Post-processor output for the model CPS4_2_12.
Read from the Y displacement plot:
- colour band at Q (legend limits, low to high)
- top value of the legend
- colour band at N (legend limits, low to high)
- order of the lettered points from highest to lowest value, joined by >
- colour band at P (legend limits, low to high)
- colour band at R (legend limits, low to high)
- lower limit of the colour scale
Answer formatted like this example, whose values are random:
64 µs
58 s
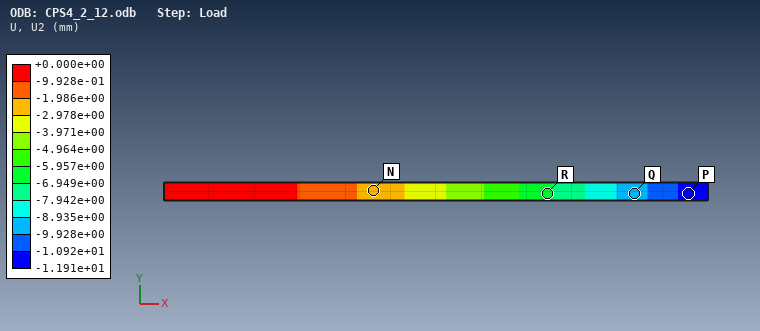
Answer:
-9.928e+00 to -8.935e+00 mm
+0.000e+00 mm
-2.978e+00 to -1.986e+00 mm
N > R > Q > P
-1.191e+01 to -1.092e+01 mm
-6.949e+00 to -5.957e+00 mm
-1.191e+01 mm
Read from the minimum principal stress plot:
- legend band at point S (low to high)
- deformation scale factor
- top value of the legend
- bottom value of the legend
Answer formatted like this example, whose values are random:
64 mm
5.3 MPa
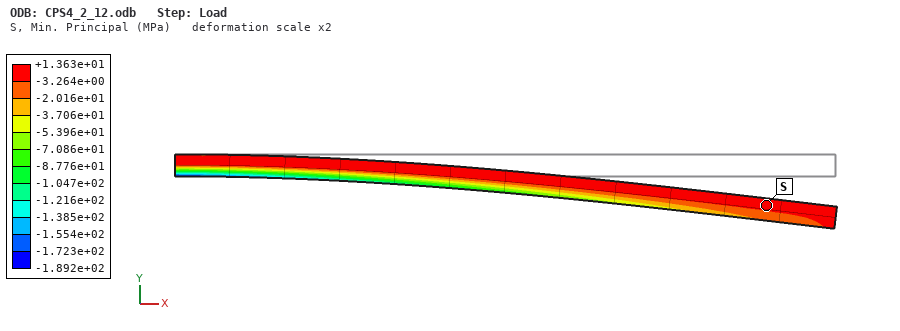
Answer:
-3.264e+00 to +1.363e+01 MPa
2
+1.363e+01 MPa
-1.892e+02 MPa
